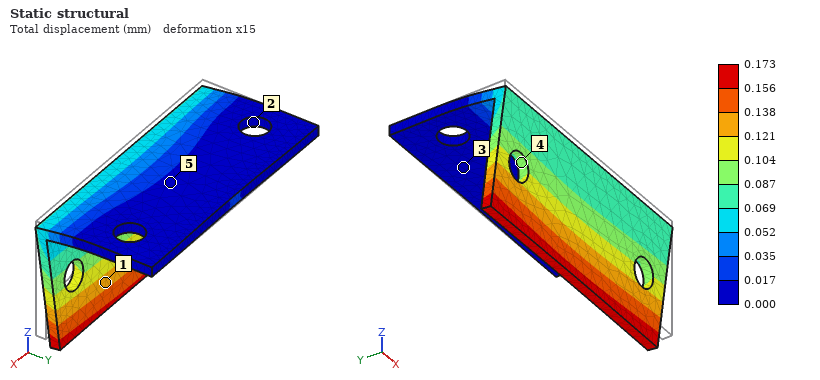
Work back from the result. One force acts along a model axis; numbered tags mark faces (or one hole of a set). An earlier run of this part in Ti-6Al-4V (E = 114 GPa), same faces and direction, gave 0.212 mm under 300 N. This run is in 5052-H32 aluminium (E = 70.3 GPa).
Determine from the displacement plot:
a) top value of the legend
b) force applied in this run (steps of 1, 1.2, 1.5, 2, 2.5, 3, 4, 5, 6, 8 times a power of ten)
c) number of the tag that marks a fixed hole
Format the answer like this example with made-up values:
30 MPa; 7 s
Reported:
0.173 mm; 150 N; 2
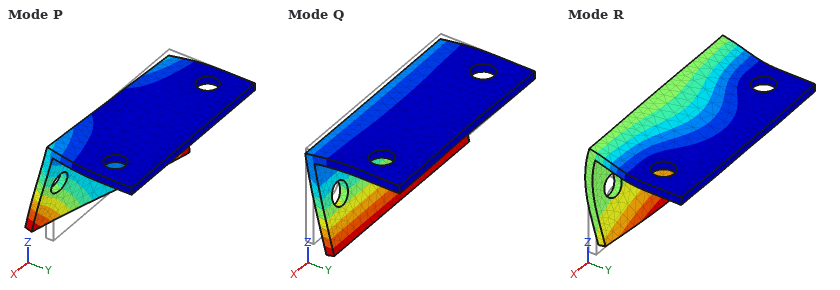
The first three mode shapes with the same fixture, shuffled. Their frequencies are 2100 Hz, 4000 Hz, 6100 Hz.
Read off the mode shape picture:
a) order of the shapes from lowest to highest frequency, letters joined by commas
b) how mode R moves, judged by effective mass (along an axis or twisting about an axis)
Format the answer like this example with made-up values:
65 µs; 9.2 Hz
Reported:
Q, P, R; along Z
